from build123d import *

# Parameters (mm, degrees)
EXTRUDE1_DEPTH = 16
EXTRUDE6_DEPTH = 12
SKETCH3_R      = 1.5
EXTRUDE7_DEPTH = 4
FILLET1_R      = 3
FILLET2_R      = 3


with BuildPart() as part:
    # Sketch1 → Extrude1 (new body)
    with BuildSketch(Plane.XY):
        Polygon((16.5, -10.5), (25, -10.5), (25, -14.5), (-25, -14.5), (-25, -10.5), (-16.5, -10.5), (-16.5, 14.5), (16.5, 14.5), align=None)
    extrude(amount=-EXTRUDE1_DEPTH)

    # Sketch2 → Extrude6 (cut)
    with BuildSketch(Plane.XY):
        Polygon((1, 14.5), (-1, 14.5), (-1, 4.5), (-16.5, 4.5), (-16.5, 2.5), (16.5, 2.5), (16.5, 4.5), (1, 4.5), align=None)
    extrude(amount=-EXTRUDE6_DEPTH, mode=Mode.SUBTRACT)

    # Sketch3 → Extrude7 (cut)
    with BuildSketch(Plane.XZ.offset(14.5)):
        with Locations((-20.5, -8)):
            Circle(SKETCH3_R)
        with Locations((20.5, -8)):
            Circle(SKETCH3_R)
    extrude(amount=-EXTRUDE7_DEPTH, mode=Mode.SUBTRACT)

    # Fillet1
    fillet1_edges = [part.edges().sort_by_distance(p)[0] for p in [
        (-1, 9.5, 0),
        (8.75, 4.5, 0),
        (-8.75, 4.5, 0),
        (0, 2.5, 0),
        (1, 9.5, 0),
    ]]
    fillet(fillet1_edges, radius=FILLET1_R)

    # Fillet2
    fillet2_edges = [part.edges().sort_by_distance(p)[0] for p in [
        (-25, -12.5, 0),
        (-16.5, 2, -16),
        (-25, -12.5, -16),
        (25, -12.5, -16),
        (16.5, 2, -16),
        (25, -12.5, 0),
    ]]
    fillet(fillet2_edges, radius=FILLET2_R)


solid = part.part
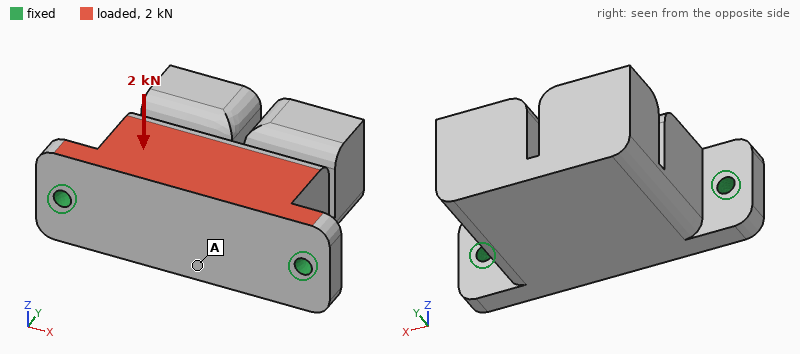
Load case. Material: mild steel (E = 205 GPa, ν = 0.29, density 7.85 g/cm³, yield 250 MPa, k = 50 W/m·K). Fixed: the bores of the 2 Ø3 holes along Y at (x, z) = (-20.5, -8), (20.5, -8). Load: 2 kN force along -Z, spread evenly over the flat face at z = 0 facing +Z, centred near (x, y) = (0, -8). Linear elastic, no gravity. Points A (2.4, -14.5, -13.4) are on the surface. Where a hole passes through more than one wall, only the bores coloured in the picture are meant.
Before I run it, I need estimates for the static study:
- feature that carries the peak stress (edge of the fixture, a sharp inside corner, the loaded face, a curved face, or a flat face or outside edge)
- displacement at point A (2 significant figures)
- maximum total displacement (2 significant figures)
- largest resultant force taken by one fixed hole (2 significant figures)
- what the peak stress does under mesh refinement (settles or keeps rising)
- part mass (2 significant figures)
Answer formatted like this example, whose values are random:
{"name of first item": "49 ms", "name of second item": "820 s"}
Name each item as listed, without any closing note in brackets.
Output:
{"feature that carries the peak stress": "edge of the fixture", "displacement at point A": "5.6 µm", "maximum total displacement": "32 µm", "largest resultant force taken by one fixed hole": "1.0 kN", "what the peak stress does under mesh refinement": "keeps rising", "part mass": "120 g"}
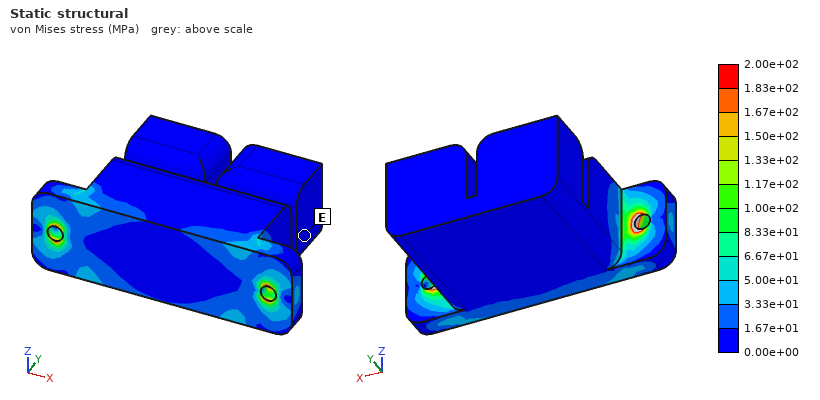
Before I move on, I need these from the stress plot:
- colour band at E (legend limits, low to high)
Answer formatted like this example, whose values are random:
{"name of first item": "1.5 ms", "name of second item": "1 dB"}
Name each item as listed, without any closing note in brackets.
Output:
{"colour band at E": "0.00e+00 to 1.67e+01 MPa"}
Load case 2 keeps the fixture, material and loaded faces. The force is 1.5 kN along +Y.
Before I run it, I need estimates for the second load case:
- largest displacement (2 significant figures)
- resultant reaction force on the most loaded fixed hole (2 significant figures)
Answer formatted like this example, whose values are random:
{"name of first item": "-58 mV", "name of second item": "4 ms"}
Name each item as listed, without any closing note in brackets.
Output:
{"largest displacement": "37 µm", "resultant reaction force on the most loaded fixed hole": "830 N"}
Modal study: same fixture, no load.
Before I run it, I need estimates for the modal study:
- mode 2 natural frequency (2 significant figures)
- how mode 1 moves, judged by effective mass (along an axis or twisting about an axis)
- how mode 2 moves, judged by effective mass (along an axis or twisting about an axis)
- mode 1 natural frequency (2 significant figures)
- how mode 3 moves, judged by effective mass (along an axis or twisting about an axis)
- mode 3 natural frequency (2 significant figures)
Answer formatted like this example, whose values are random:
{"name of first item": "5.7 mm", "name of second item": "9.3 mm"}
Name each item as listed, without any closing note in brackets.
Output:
{"mode 2 natural frequency": "7700 Hz", "how mode 1 moves, judged by effective mass": "along Z", "how mode 2 moves, judged by effective mass": "along Y", "mode 1 natural frequency": "2700 Hz", "how mode 3 moves, judged by effective mass": "along X", "mode 3 natural frequency": "9100 Hz"}
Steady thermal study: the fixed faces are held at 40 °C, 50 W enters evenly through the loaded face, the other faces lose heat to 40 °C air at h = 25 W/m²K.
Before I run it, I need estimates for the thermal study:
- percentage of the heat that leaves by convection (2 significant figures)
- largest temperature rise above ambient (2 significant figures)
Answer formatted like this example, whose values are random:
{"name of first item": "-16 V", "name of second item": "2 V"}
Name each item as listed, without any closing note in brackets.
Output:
{"percentage of the heat that leaves by convection": "12 %", "largest temperature rise above ambient": "74 K"}
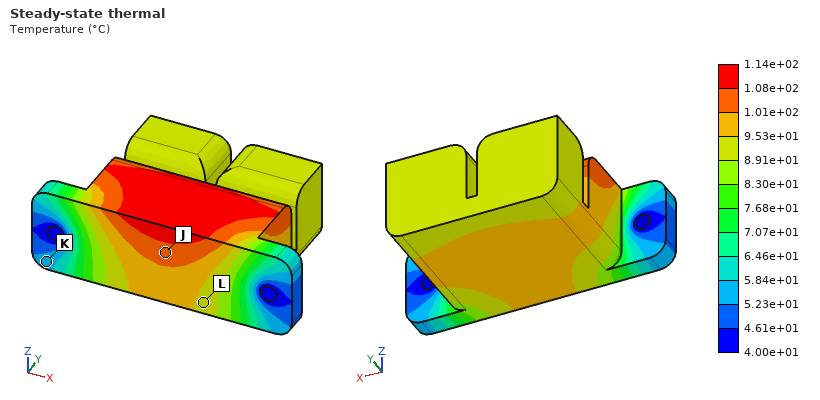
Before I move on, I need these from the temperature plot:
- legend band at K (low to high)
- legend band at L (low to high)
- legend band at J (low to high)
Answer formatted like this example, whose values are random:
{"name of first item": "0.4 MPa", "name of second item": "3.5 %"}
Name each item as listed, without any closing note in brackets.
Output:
{"legend band at K": "5.23e+01 to 5.84e+01 °C", "legend band at L": "8.91e+01 to 9.53e+01 °C", "legend band at J": "1.01e+02 to 1.08e+02 °C"}
